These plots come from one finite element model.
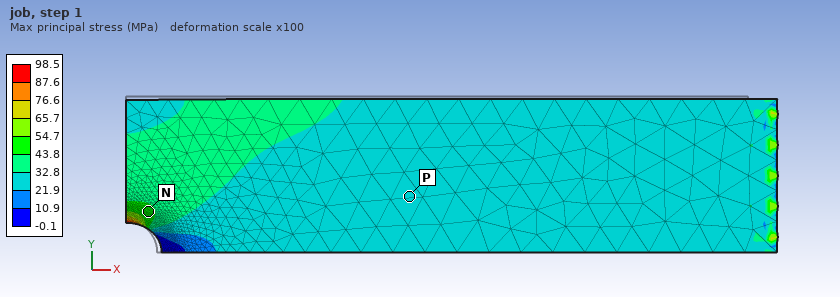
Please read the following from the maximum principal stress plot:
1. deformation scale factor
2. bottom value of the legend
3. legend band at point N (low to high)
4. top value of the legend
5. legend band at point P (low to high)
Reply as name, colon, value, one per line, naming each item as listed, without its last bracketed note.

deformation scale factor: 100
bottom value of the legend: -0.1 MPa
legend band at point N: 43.8 to 54.7 MPa
top value of the legend: 98.5 MPa
legend band at point P: 21.9 to 32.8 MPa
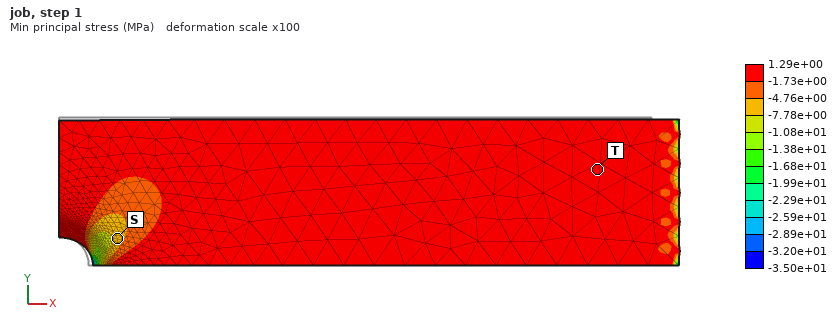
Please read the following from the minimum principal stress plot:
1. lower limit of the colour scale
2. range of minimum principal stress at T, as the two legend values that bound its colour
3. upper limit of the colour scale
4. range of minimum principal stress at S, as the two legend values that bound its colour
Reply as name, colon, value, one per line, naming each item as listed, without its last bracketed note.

lower limit of the colour scale: -3.50e+01 MPa
range of minimum principal stress at T, as the two legend values that bound its colour: -1.73e+00 to 1.29e+00 MPa
upper limit of the colour scale: 1.29e+00 MPa
range of minimum principal stress at S, as the two legend values that bound its colour: -7.78e+00 to -4.76e+00 MPa
